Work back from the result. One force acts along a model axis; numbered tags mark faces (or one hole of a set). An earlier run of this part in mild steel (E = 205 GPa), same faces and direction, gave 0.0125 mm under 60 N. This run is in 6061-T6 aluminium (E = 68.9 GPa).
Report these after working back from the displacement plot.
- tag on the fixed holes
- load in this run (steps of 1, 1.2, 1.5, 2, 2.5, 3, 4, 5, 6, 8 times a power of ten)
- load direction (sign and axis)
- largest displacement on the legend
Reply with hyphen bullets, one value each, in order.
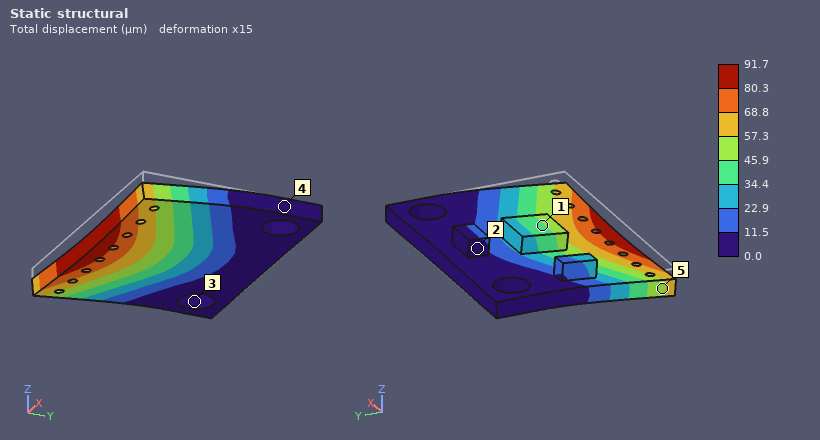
- 3
- 150 N
- -Z
- 91.7 µm
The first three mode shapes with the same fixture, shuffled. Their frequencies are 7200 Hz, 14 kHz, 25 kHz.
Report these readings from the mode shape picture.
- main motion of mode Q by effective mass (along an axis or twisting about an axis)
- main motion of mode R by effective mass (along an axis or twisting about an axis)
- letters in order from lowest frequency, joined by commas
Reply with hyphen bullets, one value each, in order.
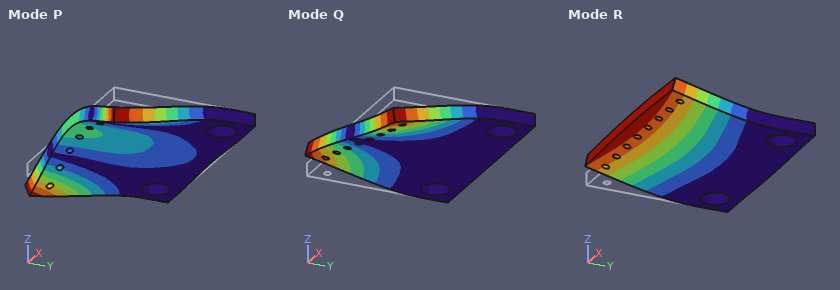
- twisting about Y
- along Z
- R, Q, P
